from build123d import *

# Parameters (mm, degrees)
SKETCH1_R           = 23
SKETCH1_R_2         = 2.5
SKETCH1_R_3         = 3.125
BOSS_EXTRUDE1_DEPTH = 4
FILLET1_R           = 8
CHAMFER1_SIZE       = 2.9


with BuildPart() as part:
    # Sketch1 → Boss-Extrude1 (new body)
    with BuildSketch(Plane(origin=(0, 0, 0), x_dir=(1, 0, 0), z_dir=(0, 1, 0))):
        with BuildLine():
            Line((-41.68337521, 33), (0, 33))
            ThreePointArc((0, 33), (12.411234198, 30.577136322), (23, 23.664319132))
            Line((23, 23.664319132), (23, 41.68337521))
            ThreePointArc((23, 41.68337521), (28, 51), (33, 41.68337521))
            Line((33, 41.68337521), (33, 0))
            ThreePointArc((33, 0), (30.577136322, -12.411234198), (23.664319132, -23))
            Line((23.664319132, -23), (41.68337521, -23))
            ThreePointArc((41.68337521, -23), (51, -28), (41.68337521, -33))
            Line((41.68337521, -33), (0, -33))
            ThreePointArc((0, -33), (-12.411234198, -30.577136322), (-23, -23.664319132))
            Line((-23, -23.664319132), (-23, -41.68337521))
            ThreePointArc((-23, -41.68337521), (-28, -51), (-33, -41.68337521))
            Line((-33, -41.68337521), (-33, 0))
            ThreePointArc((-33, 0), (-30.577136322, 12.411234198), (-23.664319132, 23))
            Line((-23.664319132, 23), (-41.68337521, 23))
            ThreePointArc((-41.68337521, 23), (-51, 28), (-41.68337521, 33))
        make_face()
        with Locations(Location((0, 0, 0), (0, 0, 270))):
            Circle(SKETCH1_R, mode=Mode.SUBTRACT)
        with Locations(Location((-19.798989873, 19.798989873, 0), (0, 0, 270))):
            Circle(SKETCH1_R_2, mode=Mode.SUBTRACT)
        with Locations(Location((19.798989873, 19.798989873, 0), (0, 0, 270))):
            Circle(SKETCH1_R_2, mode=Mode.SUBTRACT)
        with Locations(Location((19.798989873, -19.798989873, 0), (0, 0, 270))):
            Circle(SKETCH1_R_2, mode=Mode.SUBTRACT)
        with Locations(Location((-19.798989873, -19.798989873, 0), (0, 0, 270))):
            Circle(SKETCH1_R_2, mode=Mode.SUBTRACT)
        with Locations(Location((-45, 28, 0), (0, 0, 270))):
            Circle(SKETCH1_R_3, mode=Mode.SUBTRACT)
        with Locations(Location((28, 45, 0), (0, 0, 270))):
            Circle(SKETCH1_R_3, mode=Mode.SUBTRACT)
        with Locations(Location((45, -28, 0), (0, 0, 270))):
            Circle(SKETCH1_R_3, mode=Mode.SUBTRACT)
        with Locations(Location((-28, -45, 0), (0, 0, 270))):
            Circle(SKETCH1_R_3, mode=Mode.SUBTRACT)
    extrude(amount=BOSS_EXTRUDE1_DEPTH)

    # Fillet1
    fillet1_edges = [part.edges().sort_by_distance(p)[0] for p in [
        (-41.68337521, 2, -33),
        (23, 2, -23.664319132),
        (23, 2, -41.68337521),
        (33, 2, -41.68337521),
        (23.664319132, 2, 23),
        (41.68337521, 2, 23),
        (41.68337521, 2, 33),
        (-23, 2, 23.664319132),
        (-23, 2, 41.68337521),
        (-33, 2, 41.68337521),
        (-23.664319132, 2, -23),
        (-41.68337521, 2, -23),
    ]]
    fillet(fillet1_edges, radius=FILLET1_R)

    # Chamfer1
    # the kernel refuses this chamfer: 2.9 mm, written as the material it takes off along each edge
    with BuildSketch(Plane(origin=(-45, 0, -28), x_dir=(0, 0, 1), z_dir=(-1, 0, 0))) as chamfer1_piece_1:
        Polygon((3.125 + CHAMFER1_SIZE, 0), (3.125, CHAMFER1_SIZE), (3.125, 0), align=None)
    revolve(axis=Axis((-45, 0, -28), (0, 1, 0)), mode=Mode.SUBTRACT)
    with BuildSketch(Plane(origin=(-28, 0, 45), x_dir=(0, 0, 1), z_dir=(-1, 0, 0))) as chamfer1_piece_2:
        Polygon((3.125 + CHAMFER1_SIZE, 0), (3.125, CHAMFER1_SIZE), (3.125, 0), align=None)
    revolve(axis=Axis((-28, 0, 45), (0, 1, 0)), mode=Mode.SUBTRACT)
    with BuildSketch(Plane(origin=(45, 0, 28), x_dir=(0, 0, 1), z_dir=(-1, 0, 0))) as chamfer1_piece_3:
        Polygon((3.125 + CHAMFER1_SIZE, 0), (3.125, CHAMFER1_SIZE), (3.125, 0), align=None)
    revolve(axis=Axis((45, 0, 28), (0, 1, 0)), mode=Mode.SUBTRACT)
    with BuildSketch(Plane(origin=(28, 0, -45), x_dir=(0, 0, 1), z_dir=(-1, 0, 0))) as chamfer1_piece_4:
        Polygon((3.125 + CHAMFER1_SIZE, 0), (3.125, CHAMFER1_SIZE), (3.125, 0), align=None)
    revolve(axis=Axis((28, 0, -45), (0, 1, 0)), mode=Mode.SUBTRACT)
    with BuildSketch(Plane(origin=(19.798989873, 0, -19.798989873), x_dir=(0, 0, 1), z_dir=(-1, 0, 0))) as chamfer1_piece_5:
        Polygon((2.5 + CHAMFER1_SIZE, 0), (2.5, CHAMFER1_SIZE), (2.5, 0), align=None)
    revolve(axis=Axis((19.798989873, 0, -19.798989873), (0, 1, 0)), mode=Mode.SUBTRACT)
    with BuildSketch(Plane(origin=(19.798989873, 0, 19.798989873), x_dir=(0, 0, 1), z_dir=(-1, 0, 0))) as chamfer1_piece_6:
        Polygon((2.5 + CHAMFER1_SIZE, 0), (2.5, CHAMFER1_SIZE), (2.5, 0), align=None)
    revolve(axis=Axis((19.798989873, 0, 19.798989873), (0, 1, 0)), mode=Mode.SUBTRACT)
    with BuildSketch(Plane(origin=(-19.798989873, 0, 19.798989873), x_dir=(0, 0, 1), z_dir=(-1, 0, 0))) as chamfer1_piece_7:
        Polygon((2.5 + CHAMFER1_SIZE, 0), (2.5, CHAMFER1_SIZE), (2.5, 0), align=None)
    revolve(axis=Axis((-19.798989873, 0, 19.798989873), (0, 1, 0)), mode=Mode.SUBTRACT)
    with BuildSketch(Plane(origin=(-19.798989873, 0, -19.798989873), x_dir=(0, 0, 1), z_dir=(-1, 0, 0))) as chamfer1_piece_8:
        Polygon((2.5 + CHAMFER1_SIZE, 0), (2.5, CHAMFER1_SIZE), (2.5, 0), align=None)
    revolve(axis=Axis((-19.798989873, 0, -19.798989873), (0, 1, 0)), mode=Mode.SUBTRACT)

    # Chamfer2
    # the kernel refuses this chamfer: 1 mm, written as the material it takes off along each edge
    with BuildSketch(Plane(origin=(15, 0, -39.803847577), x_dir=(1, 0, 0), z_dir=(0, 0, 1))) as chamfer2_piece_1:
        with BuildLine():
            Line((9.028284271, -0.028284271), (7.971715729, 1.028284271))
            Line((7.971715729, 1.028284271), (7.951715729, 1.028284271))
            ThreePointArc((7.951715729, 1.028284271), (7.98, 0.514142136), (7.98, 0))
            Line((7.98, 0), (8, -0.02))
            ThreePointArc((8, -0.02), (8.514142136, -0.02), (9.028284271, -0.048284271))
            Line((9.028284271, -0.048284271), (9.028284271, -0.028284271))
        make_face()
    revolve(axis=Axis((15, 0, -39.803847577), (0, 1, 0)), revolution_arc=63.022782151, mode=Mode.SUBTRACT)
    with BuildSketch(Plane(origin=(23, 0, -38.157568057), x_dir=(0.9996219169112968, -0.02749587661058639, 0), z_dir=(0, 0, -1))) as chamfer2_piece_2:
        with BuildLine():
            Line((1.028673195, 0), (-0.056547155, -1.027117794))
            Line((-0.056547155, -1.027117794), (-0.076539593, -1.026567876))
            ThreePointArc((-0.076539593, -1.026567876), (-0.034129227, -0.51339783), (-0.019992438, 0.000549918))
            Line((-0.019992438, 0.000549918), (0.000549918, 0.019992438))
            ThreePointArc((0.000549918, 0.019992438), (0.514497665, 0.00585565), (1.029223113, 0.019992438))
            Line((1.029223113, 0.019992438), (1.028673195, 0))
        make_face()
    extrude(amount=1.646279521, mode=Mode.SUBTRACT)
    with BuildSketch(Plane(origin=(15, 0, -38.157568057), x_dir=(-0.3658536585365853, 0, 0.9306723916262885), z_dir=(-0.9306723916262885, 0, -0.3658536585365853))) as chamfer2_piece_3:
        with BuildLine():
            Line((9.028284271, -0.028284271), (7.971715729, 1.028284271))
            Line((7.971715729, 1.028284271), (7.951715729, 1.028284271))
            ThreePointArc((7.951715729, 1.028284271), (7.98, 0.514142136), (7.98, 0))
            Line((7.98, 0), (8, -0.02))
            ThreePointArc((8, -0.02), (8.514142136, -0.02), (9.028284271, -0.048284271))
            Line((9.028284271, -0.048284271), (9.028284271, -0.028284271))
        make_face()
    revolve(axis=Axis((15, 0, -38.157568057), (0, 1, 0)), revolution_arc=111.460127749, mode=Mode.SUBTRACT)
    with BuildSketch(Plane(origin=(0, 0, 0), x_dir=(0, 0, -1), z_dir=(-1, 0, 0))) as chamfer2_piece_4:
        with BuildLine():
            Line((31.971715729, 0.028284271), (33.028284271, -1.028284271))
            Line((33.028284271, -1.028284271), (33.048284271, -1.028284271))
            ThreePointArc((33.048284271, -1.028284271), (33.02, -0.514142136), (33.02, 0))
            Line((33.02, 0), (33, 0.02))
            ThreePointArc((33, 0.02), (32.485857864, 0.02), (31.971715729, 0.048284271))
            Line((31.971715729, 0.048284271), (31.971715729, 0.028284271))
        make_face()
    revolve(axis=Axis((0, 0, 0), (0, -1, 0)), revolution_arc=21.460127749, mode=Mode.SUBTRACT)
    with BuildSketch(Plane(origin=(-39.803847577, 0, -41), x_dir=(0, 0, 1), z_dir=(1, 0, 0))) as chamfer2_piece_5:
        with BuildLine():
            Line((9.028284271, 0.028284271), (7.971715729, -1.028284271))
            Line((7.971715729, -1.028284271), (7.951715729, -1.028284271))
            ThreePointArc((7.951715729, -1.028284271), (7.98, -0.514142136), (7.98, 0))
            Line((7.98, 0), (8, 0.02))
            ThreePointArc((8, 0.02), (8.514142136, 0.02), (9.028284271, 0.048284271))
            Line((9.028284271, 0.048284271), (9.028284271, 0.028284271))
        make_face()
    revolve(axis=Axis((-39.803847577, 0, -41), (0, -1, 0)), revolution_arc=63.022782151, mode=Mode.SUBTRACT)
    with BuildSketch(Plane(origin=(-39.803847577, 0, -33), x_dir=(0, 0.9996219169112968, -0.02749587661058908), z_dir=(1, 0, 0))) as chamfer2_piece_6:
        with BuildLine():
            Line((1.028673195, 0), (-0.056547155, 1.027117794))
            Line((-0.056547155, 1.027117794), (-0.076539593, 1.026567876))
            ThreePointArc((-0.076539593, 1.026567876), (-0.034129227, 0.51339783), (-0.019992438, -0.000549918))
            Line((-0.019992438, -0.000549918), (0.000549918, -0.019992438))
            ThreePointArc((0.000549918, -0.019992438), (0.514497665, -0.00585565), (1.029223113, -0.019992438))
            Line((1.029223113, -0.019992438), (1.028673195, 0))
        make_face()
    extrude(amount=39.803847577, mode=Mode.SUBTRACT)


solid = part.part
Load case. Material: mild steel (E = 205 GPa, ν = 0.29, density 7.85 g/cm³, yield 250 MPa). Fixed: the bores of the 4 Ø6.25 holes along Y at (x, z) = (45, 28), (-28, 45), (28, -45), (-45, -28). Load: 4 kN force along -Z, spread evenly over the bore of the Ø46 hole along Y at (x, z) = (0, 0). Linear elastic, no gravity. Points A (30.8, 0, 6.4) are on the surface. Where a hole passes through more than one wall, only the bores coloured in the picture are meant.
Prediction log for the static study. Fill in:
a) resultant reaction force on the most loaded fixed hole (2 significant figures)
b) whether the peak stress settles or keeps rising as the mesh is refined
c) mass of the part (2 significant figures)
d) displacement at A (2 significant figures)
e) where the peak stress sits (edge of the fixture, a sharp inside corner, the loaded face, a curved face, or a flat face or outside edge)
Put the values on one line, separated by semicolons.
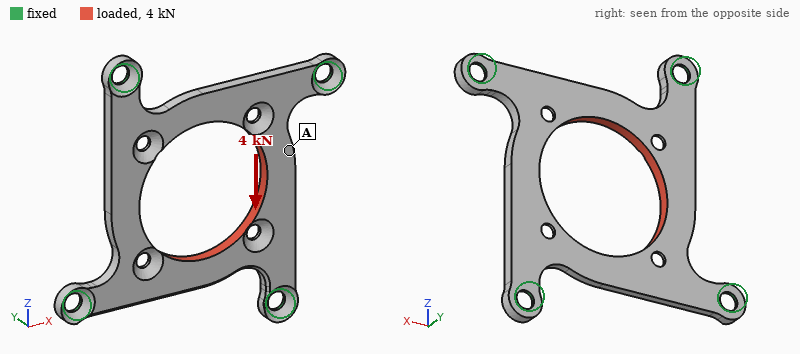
1.6 kN; keeps rising; 91 g; 9.9 µm; edge of the fixture
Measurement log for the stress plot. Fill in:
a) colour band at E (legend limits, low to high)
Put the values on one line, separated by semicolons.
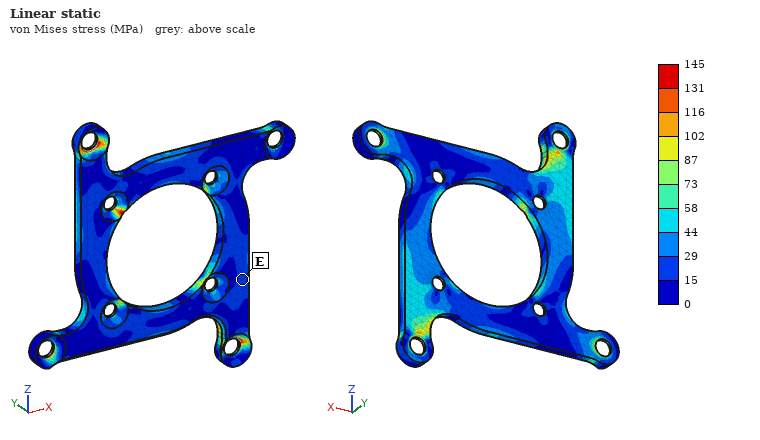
15 to 29 MPa
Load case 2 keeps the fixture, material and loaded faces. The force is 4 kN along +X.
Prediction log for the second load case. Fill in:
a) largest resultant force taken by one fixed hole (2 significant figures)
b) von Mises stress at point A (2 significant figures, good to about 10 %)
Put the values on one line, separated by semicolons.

1.6 kN; 21 MPa
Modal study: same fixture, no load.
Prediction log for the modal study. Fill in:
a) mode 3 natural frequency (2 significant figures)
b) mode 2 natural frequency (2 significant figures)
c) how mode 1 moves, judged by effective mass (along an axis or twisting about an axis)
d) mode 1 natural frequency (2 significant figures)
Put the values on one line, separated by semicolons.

3100 Hz; 3100 Hz; along Y; 2000 Hz
